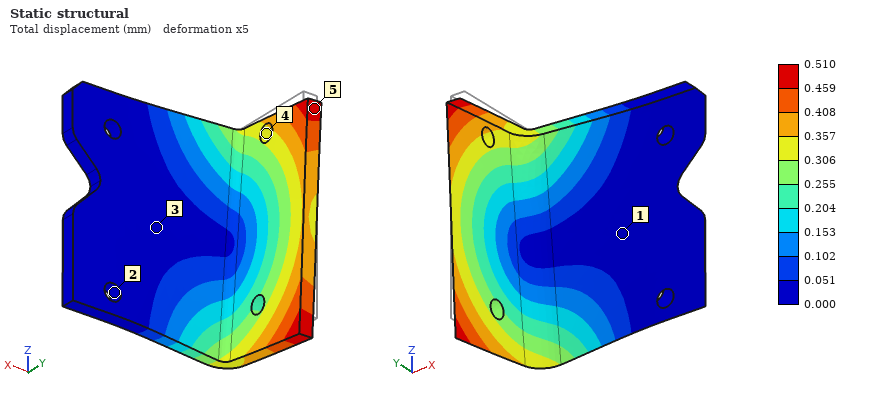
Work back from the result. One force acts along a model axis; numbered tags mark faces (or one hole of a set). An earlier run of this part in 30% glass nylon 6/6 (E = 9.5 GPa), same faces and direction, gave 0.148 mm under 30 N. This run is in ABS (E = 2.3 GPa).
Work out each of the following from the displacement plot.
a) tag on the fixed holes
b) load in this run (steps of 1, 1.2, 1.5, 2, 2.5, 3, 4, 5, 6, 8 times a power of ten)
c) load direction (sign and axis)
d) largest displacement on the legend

2
25 N
-Z
0.510 mm
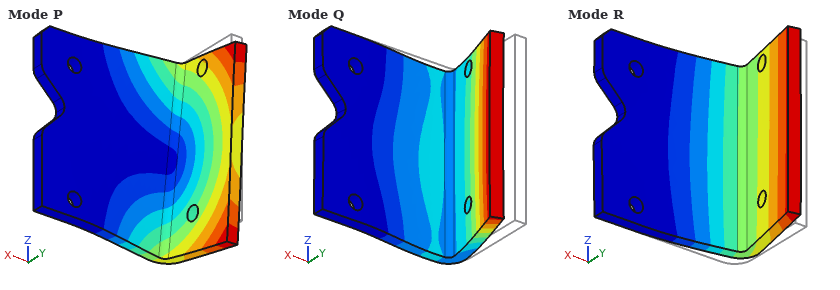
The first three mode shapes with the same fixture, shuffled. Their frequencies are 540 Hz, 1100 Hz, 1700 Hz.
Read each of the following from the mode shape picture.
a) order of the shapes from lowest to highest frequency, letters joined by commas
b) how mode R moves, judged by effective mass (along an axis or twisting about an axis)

R, P, Q
along Y
